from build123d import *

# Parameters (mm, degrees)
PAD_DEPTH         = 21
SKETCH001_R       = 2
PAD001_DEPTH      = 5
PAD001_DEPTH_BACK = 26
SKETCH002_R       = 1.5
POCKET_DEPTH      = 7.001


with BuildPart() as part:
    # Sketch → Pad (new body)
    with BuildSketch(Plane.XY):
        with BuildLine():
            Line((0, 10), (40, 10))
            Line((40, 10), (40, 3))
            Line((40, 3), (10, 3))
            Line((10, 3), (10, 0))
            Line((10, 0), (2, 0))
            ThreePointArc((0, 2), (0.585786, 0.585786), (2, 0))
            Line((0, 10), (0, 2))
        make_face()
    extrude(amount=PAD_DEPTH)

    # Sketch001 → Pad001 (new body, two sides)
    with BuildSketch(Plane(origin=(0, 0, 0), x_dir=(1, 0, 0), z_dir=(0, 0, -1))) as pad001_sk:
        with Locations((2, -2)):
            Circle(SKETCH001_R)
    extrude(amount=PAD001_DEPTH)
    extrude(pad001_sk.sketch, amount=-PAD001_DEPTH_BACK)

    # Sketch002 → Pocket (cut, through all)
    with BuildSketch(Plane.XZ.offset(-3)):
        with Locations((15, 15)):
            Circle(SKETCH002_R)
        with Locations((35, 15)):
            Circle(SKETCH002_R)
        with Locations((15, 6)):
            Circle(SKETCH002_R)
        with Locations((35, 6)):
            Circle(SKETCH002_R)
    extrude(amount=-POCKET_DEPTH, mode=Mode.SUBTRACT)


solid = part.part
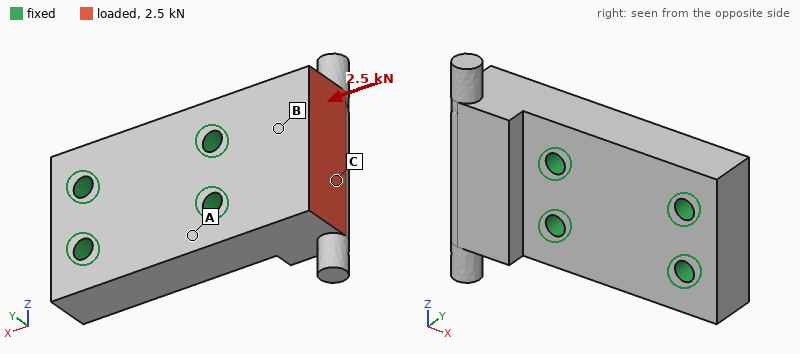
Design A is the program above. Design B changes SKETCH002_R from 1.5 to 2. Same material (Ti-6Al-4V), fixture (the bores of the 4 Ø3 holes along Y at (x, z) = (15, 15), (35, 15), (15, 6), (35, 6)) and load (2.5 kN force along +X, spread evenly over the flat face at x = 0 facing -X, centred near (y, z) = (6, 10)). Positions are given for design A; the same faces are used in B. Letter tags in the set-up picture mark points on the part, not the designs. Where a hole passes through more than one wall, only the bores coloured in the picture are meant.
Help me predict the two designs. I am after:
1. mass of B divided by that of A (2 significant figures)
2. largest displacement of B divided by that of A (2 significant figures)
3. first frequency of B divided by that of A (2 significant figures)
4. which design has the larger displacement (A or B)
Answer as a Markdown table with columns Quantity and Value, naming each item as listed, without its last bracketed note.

| Quantity | Value |
|---|---|
| mass of B divided by that of A | 0.98 |
| largest displacement of B divided by that of A | 0.92 |
| first frequency of B divided by that of A | 1.1 |
| which design has the larger displacement | A |
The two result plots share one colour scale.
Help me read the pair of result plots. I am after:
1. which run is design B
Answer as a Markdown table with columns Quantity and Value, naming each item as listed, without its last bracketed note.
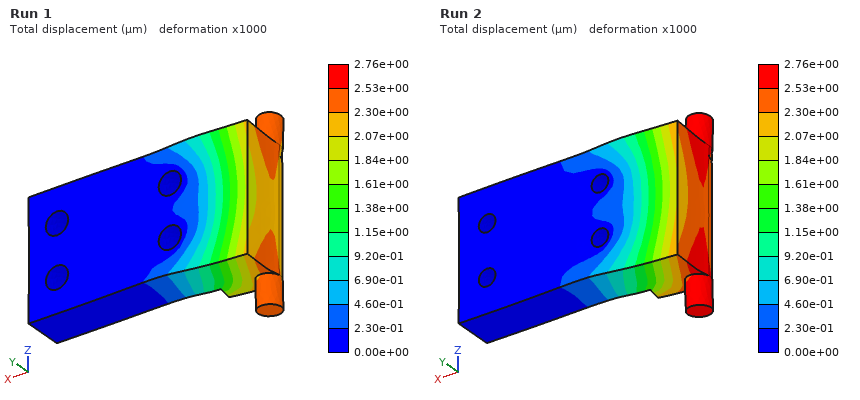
| Quantity | Value |
|---|---|
| which run is design B | Run 1 |
